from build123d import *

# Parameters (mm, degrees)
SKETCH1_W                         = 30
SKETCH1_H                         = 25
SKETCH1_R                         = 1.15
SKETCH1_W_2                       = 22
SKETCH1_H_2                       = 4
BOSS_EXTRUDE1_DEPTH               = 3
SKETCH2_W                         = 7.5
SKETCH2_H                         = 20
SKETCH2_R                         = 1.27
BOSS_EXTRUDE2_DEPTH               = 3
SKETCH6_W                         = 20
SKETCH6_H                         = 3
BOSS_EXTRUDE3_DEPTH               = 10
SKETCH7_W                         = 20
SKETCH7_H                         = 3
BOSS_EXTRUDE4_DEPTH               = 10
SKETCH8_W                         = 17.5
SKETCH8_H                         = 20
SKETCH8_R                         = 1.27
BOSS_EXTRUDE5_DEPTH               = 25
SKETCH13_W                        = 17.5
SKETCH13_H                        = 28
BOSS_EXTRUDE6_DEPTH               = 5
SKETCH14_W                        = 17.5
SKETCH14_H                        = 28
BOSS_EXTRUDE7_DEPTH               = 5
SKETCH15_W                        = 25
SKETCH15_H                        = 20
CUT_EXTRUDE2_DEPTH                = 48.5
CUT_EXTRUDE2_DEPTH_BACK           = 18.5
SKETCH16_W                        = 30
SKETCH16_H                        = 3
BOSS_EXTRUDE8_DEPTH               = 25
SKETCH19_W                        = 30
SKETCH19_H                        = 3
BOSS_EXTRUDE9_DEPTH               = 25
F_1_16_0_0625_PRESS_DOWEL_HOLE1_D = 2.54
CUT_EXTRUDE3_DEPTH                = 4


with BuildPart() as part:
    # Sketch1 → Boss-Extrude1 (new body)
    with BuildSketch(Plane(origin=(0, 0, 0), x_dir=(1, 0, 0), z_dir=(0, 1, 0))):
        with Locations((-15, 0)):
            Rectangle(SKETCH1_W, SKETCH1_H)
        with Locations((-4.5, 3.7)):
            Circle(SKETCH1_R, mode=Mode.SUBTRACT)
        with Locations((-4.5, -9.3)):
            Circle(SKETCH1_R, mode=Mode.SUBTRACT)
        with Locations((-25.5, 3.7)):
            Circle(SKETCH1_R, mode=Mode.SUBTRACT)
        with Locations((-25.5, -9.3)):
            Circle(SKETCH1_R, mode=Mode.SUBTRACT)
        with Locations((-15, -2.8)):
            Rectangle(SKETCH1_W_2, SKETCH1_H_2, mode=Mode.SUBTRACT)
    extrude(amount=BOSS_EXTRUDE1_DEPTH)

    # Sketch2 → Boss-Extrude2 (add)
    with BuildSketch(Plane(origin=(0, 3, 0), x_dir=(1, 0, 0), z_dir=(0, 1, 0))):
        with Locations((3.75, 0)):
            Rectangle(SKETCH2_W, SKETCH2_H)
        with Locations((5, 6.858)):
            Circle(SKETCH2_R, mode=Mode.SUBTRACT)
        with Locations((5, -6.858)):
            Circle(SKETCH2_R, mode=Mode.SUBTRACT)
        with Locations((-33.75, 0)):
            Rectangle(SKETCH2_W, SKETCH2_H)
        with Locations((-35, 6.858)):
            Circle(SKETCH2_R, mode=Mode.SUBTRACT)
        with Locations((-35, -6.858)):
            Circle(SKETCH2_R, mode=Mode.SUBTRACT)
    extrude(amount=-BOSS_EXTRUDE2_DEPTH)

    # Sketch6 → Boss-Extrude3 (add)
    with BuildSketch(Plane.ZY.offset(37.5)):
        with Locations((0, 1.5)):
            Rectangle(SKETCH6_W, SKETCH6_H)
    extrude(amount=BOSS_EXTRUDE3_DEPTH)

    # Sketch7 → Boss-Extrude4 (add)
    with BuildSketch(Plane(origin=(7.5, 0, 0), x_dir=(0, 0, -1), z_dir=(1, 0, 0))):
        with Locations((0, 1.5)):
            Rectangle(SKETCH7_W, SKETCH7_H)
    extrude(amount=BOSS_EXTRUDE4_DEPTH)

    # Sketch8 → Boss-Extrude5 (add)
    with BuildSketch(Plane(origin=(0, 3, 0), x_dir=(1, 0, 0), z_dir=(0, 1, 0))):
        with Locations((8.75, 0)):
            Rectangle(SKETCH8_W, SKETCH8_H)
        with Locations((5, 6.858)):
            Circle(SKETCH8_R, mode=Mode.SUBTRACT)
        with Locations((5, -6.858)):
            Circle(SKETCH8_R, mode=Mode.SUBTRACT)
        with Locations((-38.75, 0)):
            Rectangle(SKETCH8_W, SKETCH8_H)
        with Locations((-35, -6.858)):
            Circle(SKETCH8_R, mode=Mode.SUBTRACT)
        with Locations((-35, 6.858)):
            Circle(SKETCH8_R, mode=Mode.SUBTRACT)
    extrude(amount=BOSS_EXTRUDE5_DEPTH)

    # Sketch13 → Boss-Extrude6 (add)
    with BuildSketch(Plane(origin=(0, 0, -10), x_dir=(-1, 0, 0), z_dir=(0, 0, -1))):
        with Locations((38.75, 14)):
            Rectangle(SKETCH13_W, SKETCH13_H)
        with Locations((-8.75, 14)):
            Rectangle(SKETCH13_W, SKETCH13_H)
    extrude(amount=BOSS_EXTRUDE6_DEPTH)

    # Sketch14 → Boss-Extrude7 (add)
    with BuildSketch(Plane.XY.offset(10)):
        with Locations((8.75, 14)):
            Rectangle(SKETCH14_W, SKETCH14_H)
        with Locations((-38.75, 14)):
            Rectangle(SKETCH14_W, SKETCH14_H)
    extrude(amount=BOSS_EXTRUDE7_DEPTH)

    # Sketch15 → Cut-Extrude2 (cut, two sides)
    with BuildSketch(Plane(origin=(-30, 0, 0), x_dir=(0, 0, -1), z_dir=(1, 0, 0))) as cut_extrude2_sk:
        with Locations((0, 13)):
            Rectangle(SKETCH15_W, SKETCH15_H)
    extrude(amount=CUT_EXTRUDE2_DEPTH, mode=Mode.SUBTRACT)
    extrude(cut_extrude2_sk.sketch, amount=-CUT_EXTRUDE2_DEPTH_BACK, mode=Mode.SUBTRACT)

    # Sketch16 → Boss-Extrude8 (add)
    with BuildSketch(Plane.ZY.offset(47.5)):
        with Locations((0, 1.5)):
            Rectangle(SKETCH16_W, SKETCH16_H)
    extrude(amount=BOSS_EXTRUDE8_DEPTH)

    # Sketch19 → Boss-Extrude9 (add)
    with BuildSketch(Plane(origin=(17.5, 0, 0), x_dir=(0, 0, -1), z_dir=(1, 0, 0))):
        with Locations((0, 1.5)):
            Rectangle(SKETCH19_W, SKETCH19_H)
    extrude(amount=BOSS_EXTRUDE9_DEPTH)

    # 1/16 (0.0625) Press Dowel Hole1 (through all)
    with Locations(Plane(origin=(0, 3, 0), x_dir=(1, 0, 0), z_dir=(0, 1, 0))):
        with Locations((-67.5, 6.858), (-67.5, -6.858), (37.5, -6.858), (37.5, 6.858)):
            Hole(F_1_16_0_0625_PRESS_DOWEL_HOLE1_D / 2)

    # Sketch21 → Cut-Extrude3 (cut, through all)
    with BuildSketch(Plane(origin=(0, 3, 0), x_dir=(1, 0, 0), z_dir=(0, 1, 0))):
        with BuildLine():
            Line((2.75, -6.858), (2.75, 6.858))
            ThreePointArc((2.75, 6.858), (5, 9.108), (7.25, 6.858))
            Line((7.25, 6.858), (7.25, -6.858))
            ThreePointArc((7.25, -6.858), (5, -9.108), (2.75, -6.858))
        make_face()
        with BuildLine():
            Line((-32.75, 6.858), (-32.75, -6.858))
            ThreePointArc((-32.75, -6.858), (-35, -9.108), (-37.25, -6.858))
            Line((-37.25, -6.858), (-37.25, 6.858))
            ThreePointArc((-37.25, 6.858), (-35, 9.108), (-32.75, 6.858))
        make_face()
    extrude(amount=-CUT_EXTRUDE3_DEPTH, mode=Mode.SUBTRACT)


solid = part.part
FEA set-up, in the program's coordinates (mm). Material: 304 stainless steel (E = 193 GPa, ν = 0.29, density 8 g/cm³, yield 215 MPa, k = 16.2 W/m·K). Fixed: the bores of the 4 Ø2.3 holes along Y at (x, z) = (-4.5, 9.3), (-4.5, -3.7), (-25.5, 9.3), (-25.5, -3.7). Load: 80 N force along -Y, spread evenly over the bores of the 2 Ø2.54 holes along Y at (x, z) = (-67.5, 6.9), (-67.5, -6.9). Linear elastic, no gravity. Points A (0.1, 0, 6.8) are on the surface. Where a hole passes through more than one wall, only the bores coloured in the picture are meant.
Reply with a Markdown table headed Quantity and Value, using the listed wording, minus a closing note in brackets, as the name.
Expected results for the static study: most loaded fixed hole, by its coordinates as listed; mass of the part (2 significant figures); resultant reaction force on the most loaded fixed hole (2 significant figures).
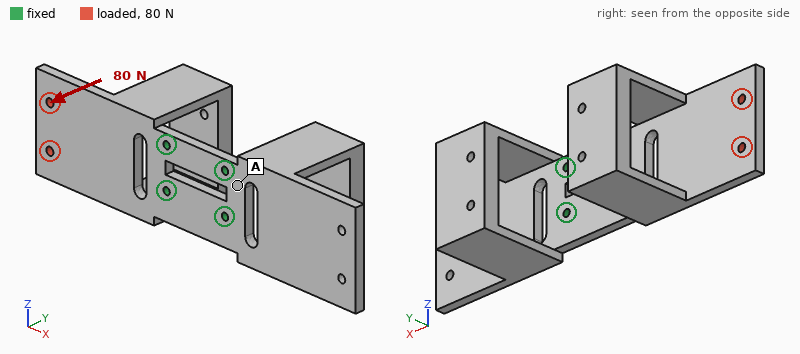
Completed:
| Quantity | Value |
|---|---|
| most loaded fixed hole, by its coordinates as listed | (-25.5, -3.7) |
| mass of the part | 140 g |
| resultant reaction force on the most loaded fixed hole | 84 N |
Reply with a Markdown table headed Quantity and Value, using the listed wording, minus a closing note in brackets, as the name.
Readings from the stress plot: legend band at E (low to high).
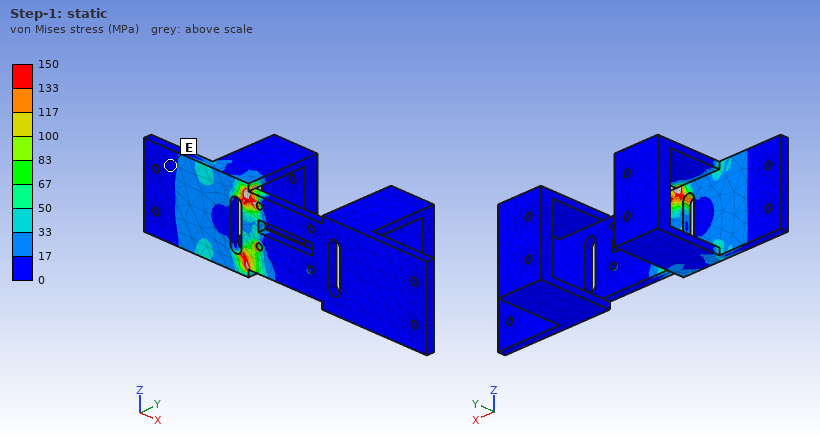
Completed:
| Quantity | Value |
|---|---|
| legend band at E | 0 to 17 MPa |
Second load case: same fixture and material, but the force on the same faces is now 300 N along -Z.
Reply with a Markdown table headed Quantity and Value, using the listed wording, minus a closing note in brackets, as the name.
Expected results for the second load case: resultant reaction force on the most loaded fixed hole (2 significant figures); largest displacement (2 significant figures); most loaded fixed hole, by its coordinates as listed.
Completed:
| Quantity | Value |
|---|---|
| resultant reaction force on the most loaded fixed hole | 660 N |
| largest displacement | 23 µm |
| most loaded fixed hole, by its coordinates as listed | (-25.5, 9.3) |
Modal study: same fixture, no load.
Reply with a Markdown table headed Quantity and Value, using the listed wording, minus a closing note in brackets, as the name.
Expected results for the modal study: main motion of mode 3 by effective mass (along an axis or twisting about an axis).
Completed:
| Quantity | Value |
|---|---|
| main motion of mode 3 by effective mass | along Z |
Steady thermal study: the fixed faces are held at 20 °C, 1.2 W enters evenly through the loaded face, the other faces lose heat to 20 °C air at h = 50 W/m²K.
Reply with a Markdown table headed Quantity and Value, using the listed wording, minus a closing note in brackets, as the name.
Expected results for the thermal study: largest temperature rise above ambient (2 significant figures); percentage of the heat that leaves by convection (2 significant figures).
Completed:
| Quantity | Value |
|---|---|
| largest temperature rise above ambient | 15 K |
| percentage of the heat that leaves by convection | 91 % |
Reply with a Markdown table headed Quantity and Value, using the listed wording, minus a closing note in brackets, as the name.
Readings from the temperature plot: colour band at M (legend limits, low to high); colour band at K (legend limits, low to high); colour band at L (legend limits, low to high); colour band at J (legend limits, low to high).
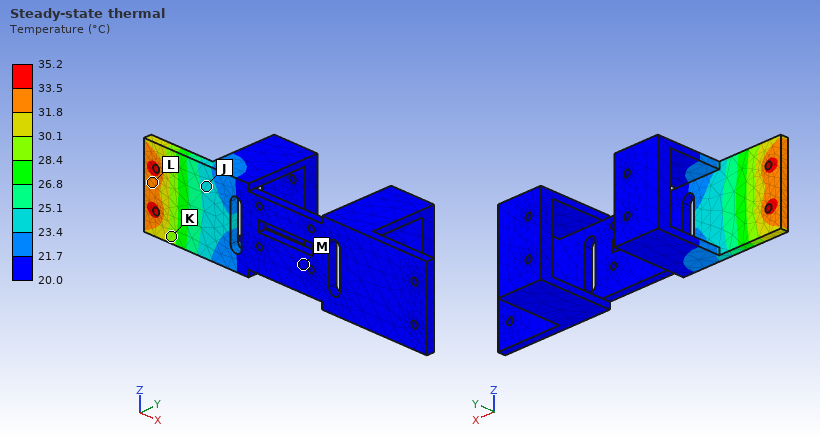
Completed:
| Quantity | Value |
|---|---|
| colour band at M | 20.0 to 21.7 °C |
| colour band at K | 28.4 to 30.1 °C |
| colour band at L | 31.8 to 33.5 °C |
| colour band at J | 23.4 to 25.1 °C |
